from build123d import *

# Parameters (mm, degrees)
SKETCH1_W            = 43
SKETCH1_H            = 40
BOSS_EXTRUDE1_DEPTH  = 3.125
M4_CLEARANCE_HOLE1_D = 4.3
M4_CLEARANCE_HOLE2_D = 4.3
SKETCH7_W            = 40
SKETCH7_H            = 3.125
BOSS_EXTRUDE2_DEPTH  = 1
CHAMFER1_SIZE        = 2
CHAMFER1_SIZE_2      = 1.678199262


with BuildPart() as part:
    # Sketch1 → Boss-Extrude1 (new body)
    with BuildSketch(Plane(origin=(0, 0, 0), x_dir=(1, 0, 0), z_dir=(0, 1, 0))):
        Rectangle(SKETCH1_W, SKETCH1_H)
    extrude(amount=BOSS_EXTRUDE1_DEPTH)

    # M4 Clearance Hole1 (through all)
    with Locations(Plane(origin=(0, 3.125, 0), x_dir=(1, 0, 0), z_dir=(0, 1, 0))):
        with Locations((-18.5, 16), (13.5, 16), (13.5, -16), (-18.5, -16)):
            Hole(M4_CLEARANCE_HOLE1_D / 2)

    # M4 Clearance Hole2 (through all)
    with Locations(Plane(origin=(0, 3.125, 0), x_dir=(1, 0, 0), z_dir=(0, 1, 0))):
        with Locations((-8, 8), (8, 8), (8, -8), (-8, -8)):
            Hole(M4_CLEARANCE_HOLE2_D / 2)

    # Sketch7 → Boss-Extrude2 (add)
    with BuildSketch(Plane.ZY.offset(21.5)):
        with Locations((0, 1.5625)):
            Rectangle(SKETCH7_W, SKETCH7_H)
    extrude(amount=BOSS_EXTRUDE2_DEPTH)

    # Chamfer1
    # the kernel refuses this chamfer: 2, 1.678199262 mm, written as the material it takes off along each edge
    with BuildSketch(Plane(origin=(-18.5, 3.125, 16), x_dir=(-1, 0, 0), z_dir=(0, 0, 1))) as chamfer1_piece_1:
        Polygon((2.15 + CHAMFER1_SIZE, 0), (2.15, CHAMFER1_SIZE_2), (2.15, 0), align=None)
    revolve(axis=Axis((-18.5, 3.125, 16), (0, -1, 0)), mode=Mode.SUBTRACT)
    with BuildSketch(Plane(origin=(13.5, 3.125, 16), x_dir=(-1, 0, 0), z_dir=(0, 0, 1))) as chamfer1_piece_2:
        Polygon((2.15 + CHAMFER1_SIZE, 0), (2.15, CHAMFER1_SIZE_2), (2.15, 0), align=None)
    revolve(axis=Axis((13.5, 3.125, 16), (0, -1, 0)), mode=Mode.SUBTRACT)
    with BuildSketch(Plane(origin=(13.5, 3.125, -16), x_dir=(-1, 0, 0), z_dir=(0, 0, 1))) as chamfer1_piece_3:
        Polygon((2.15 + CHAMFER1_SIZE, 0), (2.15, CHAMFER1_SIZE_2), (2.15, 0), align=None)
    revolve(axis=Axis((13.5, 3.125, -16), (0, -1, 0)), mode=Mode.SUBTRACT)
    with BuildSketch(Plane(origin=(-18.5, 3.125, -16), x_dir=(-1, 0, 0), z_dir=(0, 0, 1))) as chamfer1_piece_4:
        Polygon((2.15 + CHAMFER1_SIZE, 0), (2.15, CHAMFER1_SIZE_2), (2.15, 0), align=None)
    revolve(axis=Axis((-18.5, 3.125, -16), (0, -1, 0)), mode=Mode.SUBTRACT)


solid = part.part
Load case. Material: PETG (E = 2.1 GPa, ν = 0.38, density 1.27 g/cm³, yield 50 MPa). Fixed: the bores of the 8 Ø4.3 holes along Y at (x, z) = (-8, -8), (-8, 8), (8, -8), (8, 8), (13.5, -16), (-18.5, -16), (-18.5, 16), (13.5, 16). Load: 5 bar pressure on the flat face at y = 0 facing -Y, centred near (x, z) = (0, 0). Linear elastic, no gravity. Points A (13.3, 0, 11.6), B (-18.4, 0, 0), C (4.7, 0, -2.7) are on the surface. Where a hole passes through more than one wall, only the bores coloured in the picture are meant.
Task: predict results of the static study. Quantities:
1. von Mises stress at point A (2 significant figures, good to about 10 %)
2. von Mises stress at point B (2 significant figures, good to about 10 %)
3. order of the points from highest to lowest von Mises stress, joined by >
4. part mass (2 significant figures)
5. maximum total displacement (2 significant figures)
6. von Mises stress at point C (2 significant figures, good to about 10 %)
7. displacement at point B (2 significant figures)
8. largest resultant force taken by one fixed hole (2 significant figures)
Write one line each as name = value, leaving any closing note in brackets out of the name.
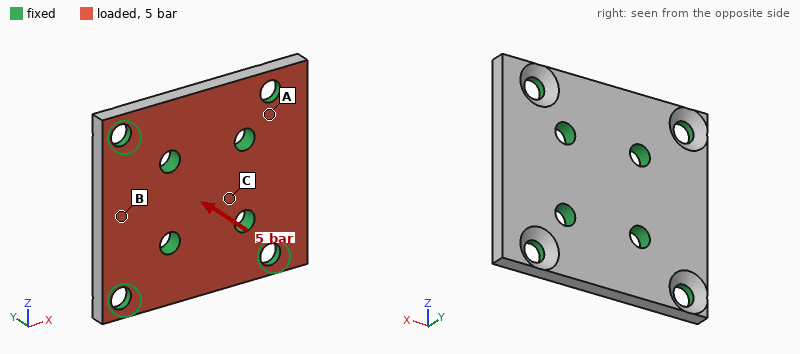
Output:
von Mises stress at point A = 9.3 MPa
von Mises stress at point B = 4.6 MPa
order of the points from highest to lowest von Mises stress, joined by > = A > B > C
part mass = 6.4 g
maximum total displacement = 0.22 mm
von Mises stress at point C = 2.5 MPa
displacement at point B = 0.12 mm
largest resultant force taken by one fixed hole = 140 N
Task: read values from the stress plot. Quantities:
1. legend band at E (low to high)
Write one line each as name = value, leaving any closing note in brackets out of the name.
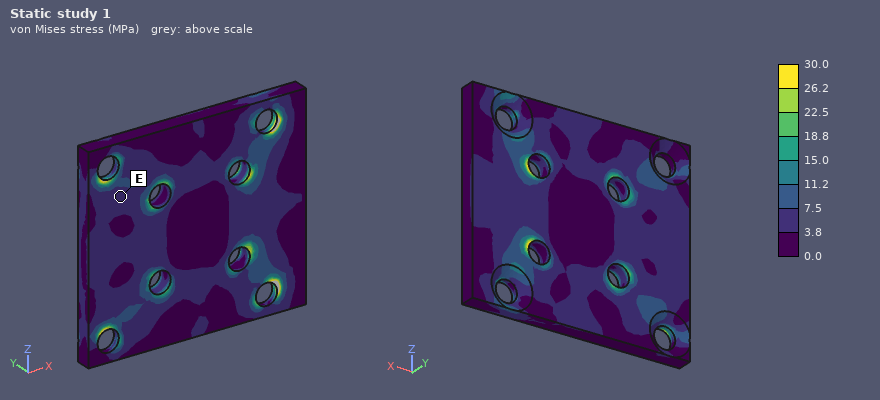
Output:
legend band at E = 3.8 to 7.5 MPa
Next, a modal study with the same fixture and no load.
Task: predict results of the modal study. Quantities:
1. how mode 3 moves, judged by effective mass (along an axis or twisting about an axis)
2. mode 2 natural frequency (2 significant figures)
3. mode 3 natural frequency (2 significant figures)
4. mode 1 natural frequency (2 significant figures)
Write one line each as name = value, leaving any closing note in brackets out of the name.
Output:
how mode 3 moves, judged by effective mass = twisting about X
mode 2 natural frequency = 5500 Hz
mode 3 natural frequency = 6700 Hz
mode 1 natural frequency = 5000 Hz
